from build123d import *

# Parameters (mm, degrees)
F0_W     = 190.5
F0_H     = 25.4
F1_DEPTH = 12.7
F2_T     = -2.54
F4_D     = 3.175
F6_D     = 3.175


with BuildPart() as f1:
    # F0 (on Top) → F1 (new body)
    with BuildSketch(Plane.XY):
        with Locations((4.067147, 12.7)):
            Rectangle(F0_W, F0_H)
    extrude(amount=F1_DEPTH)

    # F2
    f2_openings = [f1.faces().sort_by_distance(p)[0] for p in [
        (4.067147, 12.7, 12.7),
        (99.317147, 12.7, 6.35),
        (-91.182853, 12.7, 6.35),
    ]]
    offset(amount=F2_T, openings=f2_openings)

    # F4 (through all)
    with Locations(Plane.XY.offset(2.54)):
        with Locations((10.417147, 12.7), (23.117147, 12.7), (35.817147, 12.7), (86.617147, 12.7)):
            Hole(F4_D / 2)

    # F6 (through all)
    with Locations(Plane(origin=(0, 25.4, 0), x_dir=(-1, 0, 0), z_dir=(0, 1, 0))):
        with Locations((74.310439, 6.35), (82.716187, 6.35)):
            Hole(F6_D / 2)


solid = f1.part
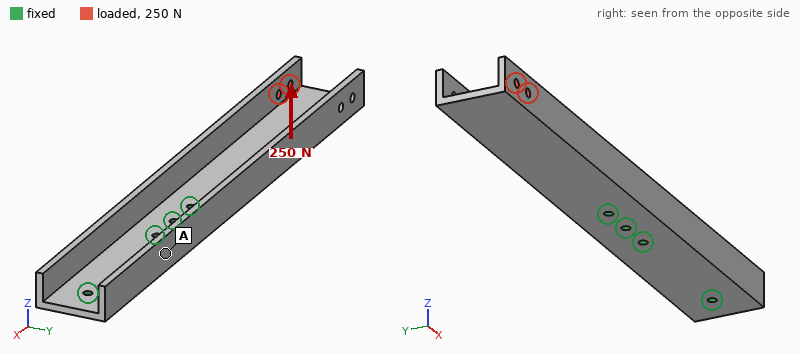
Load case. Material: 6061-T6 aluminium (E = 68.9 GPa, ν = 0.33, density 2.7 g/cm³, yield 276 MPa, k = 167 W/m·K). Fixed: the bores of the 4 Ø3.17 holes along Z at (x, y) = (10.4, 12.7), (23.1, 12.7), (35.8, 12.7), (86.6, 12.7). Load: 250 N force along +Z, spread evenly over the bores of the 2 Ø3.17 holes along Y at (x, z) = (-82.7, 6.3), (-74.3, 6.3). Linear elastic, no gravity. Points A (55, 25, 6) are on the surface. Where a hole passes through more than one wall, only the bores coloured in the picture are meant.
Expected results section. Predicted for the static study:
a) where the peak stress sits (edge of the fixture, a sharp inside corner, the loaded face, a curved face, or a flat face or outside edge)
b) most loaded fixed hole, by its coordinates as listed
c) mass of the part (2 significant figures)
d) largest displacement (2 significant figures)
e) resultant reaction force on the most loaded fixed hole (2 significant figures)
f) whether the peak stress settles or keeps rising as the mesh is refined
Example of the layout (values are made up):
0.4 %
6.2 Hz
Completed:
edge of the fixture
(10.4, 12.7)
59 g
1.5 mm
1.3 kN
keeps rising
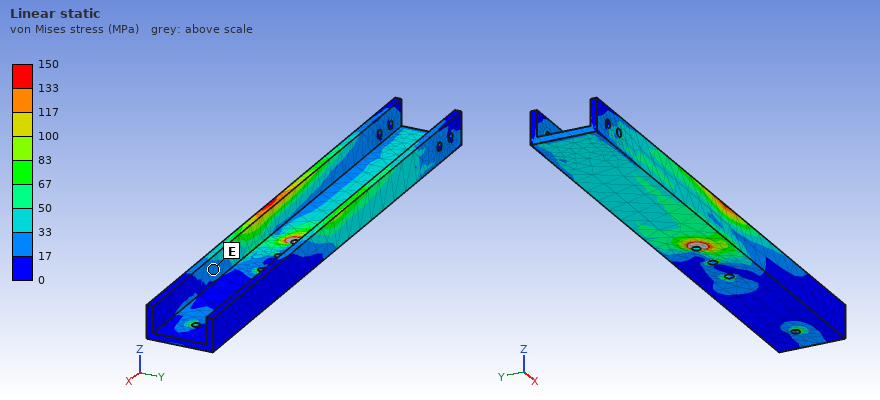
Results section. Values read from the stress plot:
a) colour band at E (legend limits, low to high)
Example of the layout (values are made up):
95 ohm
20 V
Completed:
17 to 33 MPa
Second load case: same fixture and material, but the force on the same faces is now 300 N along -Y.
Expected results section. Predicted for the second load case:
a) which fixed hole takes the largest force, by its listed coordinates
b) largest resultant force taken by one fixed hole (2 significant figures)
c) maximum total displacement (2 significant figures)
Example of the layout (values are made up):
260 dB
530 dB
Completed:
(10.4, 12.7)
1.2 kN
0.73 mm
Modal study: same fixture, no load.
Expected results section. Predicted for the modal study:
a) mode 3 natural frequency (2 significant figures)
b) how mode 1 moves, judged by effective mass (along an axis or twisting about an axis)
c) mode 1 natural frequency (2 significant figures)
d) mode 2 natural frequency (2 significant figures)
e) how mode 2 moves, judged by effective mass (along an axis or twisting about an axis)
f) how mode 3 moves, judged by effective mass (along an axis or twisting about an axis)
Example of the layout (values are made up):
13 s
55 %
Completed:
1900 Hz
along Z
750 Hz
1100 Hz
along Y
along Y
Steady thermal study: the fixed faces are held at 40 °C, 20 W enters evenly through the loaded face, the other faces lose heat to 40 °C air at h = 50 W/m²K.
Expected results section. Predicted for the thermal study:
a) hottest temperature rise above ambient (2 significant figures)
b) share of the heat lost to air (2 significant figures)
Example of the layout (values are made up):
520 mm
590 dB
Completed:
67 K
66 %
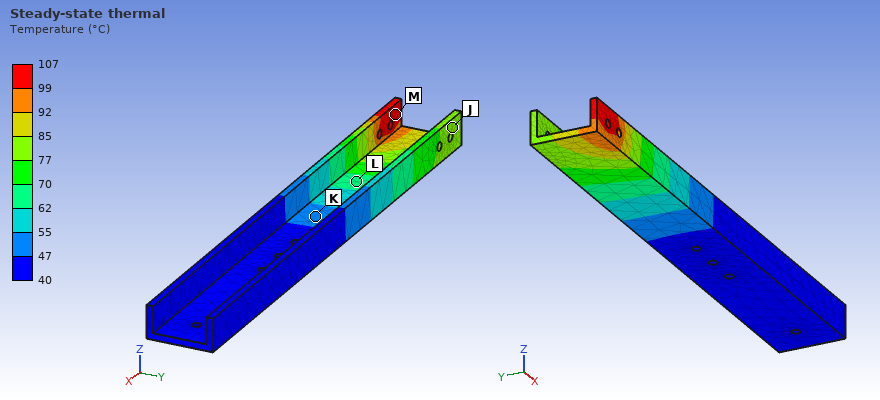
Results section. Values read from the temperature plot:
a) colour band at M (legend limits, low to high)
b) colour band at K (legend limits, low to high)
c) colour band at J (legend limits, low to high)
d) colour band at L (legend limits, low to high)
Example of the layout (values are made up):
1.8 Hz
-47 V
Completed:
99 to 107 °C
47 to 55 °C
77 to 85 °C
62 to 70 °C
